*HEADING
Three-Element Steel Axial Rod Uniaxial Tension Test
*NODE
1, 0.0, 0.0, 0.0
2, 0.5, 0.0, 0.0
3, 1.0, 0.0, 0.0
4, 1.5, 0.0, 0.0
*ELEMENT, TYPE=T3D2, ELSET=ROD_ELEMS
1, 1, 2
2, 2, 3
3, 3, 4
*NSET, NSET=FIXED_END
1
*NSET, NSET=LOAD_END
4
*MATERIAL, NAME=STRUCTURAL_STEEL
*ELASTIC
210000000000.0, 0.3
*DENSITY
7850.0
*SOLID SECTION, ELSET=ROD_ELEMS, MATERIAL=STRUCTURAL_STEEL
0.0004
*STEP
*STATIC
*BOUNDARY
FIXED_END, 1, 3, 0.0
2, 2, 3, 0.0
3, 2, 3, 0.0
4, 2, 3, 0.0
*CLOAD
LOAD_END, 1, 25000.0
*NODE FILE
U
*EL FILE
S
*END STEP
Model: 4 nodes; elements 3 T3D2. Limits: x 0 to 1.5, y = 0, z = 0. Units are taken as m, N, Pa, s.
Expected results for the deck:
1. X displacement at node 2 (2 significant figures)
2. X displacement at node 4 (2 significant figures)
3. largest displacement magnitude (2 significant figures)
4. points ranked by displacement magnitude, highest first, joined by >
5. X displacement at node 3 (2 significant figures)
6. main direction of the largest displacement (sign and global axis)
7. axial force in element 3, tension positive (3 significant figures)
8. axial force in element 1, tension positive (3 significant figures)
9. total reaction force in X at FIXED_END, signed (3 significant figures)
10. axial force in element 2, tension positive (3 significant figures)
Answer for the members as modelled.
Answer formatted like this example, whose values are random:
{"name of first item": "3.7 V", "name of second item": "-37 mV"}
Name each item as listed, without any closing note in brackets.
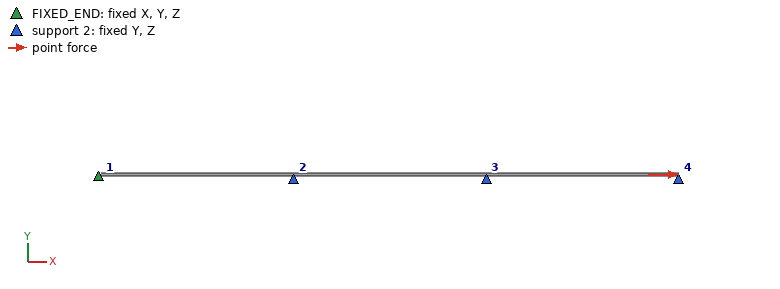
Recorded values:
{"X displacement at node 2": "1.5e-04 m", "X displacement at node 4": "4.5e-04 m", "largest displacement magnitude": "4.5e-04 m", "points ranked by displacement magnitude, highest first, joined by >": "node 4 > node 3 > node 2 > node 1", "X displacement at node 3": "3.0e-04 m", "main direction of the largest displacement": "+X", "axial force in element 3, tension positive": "25000 N", "axial force in element 1, tension positive": "25000 N", "total reaction force in X at FIXED_END, signed": "-25000 N", "axial force in element 2, tension positive": "25000 N"}
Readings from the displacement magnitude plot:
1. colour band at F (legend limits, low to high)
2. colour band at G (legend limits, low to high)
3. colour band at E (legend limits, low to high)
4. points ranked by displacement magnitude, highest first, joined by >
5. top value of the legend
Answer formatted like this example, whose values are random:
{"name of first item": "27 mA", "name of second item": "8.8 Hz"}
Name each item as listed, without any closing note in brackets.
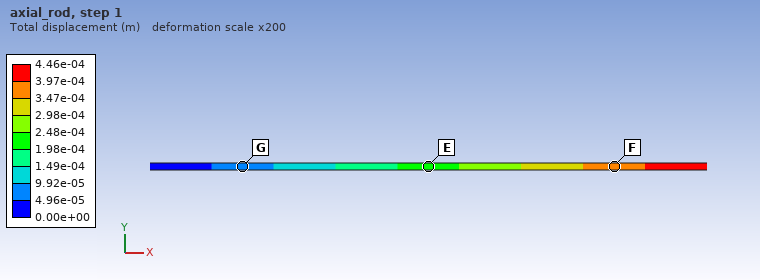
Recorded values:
{"colour band at F": "3.47e-04 to 3.97e-04 m", "colour band at G": "4.96e-05 to 9.92e-05 m", "colour band at E": "1.98e-04 to 2.48e-04 m", "points ranked by displacement magnitude, highest first, joined by >": "F > E > G", "top value of the legend": "4.46e-04 m"}
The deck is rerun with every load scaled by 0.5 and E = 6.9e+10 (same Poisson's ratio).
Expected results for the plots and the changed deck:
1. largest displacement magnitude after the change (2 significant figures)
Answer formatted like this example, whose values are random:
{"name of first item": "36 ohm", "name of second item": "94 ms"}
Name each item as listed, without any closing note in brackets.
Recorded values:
{"largest displacement magnitude after the change": "6.8e-04 m"}
